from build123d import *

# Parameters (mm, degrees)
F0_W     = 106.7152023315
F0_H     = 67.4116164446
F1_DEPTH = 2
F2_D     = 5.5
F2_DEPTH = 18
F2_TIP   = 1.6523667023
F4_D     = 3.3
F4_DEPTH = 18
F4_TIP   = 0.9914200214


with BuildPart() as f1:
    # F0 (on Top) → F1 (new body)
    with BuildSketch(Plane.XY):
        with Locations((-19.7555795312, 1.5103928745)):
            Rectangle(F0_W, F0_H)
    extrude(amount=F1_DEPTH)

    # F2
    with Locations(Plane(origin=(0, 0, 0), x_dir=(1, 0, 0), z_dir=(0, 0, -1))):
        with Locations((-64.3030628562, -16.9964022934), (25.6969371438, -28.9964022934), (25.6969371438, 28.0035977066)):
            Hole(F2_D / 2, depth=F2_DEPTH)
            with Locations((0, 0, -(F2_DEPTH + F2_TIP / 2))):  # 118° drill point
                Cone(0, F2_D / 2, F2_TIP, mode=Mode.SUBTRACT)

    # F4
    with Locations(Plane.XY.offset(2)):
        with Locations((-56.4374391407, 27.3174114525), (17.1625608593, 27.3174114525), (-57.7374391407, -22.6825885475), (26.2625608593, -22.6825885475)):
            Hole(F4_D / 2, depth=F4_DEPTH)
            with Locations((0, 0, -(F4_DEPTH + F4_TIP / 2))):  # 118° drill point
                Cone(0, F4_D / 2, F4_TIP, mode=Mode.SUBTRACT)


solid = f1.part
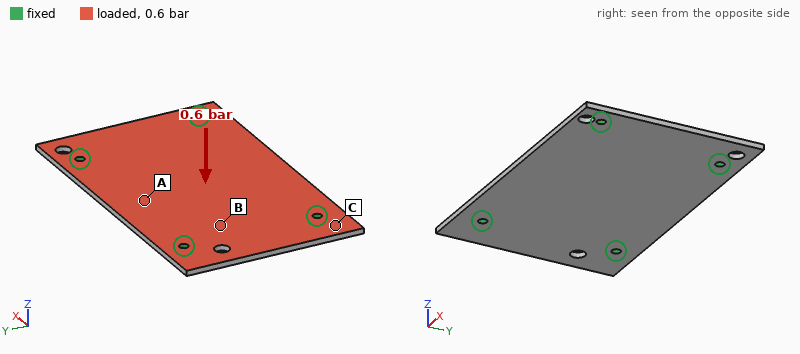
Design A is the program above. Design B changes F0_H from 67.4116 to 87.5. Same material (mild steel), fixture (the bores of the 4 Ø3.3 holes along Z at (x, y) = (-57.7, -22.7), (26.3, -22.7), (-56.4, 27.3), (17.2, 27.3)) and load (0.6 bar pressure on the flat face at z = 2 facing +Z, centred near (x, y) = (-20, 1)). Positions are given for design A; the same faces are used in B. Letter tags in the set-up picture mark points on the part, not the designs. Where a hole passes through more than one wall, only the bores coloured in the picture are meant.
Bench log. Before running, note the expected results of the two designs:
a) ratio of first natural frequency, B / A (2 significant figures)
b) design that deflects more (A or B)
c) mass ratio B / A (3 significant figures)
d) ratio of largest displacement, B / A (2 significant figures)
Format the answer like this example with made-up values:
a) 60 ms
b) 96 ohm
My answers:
a) 0.94
b) B
c) 1.30
d) 1.3
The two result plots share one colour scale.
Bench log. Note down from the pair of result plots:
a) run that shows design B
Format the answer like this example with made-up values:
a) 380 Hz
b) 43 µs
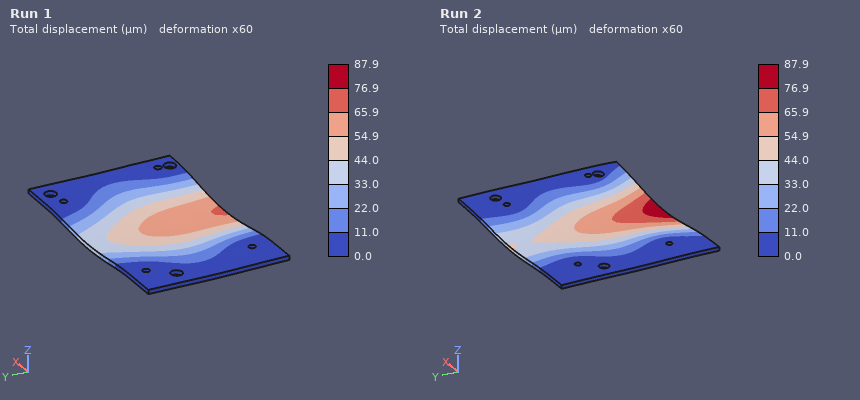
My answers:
a) Run 2
